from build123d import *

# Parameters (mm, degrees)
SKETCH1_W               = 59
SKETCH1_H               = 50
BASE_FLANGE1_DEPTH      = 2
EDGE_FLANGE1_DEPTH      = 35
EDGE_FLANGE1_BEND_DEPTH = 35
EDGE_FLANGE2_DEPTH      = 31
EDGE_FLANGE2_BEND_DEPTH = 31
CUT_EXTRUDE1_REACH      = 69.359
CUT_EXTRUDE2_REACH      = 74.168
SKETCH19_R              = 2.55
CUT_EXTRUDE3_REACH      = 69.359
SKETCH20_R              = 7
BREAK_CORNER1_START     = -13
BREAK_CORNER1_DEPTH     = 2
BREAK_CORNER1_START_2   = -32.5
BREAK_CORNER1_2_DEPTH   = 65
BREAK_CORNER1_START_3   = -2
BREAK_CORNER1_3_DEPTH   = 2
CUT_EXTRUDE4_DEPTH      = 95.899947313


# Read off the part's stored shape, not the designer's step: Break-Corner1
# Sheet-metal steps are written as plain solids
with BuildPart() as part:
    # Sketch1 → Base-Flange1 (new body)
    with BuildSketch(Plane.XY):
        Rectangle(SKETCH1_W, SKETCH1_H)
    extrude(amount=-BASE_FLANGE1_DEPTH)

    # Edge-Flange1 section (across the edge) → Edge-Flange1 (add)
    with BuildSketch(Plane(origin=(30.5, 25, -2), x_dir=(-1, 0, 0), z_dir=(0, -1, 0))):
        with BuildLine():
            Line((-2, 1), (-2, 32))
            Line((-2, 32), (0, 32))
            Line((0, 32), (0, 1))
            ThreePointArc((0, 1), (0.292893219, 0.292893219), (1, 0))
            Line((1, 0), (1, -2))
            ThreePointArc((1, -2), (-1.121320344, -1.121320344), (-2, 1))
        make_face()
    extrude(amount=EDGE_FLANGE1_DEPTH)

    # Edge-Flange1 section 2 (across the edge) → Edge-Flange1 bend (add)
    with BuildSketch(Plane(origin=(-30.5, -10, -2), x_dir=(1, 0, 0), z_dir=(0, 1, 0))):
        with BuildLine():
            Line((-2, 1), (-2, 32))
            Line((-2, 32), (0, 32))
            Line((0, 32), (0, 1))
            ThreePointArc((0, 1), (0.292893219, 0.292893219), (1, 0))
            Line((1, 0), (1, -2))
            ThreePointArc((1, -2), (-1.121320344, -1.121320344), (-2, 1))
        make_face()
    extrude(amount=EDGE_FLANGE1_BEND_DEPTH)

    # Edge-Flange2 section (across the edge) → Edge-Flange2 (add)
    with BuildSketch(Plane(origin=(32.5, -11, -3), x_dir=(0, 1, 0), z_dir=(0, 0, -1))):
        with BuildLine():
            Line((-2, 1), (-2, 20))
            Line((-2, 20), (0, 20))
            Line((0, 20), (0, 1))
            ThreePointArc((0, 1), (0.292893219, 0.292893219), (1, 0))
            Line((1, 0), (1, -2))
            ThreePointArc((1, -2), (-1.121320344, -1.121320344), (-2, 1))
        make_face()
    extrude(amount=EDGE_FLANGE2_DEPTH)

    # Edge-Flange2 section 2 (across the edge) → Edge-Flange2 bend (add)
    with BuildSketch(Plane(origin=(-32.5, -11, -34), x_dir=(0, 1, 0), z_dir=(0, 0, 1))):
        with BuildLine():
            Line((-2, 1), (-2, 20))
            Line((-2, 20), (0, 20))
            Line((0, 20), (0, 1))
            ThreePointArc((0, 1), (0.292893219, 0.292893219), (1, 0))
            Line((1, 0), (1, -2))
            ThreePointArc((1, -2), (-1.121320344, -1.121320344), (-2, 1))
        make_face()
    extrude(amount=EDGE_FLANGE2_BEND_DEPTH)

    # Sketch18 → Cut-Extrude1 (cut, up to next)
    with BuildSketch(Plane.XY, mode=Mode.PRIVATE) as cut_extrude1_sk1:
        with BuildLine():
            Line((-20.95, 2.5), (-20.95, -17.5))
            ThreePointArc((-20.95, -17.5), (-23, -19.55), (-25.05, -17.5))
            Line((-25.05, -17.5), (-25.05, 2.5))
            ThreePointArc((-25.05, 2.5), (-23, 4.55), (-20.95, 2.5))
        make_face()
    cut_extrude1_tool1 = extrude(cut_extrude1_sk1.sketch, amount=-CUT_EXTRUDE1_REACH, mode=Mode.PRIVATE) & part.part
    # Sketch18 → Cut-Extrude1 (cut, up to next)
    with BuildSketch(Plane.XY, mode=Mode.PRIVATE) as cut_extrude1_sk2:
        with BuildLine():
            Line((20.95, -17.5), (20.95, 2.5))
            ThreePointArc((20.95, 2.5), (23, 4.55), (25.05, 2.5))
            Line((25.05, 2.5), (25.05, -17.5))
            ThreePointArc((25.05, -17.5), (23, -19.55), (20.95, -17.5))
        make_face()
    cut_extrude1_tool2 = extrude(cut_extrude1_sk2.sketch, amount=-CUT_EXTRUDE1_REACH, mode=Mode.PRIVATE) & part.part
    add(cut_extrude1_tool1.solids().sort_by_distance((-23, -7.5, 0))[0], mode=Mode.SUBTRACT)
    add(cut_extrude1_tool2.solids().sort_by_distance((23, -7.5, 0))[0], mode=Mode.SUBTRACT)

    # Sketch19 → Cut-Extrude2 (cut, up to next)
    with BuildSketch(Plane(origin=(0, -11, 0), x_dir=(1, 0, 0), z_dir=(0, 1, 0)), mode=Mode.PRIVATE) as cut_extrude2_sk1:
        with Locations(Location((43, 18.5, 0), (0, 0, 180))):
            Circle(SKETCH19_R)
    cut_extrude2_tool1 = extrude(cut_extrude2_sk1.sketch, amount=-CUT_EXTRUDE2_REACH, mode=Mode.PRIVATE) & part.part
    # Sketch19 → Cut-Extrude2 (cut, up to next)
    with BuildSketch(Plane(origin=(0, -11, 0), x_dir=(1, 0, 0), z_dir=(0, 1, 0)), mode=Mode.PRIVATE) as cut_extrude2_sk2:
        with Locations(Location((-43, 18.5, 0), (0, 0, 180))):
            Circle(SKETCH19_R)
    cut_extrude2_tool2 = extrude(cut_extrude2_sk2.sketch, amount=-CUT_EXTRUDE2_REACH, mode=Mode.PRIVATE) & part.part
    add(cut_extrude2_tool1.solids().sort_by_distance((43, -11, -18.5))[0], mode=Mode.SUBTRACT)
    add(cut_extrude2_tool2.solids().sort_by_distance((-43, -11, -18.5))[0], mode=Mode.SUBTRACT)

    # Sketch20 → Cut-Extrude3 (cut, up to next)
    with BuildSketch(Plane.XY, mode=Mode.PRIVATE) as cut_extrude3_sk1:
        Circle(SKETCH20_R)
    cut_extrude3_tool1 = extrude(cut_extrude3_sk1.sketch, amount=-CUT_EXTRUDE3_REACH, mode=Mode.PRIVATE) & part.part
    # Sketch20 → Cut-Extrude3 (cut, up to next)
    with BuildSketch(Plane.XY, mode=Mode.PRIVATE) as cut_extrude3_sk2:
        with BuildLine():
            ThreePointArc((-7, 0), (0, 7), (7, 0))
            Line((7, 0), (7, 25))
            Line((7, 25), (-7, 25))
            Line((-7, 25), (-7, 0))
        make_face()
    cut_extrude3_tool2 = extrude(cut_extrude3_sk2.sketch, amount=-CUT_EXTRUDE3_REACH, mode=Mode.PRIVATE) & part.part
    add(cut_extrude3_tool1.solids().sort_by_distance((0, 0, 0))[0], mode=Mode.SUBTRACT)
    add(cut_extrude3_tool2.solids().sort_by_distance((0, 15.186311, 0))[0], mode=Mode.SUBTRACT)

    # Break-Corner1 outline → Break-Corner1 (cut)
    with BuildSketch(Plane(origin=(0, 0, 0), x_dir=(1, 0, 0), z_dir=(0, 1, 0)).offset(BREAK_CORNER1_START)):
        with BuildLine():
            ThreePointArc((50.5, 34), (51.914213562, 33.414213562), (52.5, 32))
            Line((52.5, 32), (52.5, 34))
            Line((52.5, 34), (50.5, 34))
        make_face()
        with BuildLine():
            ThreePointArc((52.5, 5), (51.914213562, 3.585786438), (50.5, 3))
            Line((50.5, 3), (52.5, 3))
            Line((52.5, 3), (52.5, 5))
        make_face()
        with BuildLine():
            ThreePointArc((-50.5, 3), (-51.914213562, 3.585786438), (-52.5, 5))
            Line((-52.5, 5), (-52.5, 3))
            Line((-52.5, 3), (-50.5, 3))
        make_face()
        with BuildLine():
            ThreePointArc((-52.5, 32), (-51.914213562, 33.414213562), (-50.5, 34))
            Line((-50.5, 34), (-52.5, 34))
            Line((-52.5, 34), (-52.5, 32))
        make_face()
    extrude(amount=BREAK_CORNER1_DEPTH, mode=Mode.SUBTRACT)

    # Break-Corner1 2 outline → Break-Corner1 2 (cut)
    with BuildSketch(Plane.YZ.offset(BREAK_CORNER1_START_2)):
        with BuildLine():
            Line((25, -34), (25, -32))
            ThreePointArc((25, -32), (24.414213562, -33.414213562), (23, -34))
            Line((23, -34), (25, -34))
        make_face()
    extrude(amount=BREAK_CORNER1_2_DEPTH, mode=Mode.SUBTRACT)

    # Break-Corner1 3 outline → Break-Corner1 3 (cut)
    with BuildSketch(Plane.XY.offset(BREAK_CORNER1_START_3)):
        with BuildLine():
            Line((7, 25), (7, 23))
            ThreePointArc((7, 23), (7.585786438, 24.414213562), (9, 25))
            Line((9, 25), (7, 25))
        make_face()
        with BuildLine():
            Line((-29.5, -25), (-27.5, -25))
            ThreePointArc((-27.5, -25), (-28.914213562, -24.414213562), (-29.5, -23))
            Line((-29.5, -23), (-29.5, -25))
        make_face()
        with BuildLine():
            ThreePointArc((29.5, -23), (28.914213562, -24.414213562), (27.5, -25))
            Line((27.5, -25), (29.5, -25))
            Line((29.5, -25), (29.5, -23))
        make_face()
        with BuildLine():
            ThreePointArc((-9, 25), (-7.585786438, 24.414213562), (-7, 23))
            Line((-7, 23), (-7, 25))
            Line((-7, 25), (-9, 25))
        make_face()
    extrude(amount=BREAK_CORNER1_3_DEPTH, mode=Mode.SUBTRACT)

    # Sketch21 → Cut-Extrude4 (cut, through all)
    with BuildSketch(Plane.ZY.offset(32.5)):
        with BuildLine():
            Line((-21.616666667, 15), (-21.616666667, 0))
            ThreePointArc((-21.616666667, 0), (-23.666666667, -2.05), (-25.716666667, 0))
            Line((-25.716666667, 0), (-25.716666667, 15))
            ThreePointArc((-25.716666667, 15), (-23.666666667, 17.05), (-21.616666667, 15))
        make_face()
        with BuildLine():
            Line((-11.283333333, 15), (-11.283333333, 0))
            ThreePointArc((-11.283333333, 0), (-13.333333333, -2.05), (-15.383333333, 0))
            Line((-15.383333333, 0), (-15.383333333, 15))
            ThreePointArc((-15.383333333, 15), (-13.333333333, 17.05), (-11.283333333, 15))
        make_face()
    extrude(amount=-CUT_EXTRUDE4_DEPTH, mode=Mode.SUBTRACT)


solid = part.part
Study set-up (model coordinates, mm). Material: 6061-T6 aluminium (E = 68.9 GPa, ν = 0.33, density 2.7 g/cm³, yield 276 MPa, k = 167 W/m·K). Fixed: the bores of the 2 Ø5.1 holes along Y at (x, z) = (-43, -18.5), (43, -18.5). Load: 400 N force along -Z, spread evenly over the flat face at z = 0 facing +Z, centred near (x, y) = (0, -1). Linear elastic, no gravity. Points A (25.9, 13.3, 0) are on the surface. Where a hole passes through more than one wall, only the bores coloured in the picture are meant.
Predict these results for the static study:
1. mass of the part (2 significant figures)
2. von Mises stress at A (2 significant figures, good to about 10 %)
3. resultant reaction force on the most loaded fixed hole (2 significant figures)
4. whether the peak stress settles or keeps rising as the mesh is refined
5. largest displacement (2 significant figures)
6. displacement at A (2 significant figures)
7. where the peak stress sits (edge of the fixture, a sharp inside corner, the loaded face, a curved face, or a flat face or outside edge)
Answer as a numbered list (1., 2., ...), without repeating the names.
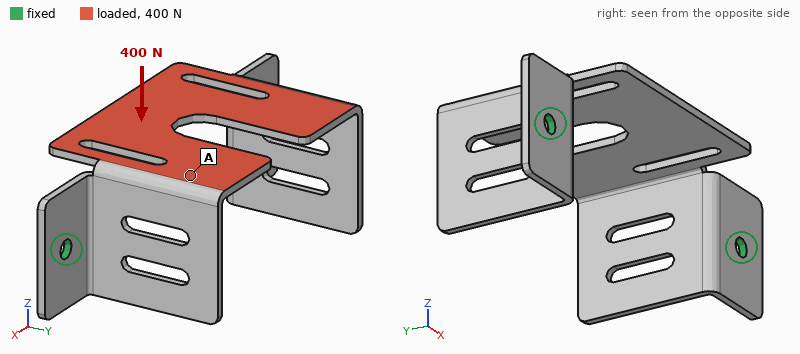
1. 31 g
2. 34 MPa
3. 230 N
4. keeps rising
5. 0.77 mm
6. 0.34 mm
7. a sharp inside corner
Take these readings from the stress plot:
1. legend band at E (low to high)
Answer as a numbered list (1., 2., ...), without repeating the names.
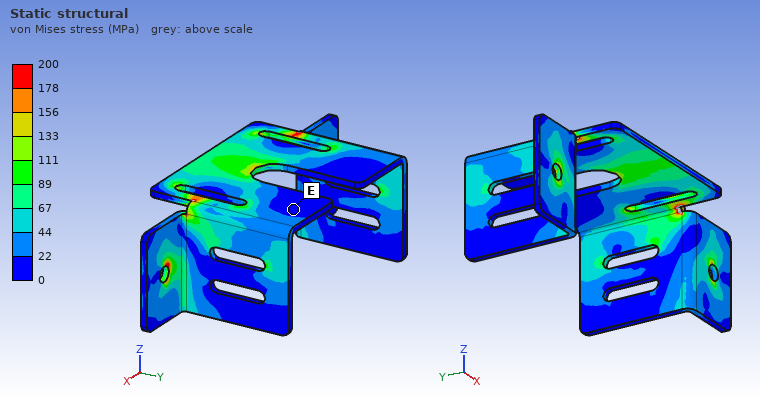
1. 0 to 22 MPa
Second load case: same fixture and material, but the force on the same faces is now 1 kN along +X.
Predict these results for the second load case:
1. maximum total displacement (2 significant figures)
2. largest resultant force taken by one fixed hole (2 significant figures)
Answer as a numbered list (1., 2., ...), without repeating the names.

1. 0.36 mm
2. 520 N
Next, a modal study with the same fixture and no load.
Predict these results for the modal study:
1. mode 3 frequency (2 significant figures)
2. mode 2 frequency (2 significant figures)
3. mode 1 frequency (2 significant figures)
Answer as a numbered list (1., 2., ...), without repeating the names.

1. 1300 Hz
2. 1100 Hz
3. 910 Hz
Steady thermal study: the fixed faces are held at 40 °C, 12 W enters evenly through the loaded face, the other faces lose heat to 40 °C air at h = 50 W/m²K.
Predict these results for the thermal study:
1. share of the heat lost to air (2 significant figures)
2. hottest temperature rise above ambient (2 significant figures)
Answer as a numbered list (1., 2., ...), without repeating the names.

1. 46 %
2. 25 K
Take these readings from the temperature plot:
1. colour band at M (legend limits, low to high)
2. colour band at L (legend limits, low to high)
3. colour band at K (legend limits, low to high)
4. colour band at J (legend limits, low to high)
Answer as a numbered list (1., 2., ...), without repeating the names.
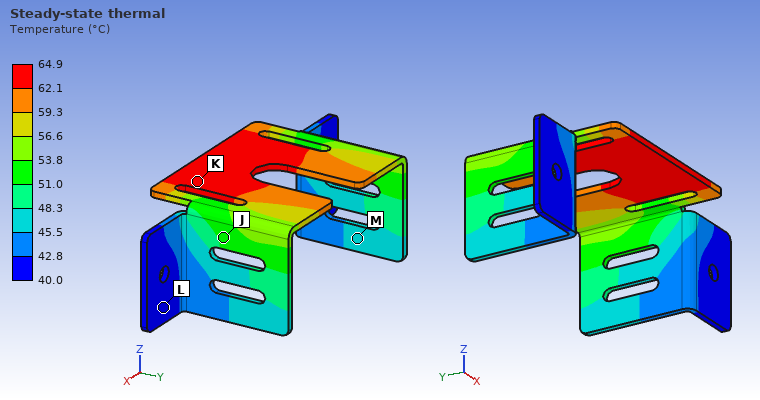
1. 45.5 to 48.3 °C
2. 40.0 to 42.8 °C
3. 62.1 to 64.9 °C
4. 51.0 to 53.8 °C
